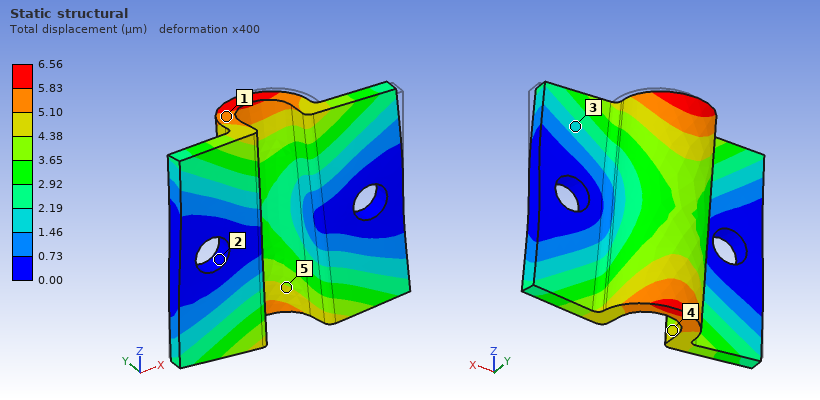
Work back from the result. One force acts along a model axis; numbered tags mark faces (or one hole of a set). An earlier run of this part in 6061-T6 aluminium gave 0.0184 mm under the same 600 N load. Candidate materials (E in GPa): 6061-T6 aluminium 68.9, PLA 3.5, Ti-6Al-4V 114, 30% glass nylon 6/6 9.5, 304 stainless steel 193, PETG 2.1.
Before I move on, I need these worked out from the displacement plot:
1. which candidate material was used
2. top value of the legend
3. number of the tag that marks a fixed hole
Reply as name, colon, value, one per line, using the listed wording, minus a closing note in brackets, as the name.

which candidate material was used: 304 stainless steel
top value of the legend: 6.56 µm
number of the tag that marks a fixed hole: 2
